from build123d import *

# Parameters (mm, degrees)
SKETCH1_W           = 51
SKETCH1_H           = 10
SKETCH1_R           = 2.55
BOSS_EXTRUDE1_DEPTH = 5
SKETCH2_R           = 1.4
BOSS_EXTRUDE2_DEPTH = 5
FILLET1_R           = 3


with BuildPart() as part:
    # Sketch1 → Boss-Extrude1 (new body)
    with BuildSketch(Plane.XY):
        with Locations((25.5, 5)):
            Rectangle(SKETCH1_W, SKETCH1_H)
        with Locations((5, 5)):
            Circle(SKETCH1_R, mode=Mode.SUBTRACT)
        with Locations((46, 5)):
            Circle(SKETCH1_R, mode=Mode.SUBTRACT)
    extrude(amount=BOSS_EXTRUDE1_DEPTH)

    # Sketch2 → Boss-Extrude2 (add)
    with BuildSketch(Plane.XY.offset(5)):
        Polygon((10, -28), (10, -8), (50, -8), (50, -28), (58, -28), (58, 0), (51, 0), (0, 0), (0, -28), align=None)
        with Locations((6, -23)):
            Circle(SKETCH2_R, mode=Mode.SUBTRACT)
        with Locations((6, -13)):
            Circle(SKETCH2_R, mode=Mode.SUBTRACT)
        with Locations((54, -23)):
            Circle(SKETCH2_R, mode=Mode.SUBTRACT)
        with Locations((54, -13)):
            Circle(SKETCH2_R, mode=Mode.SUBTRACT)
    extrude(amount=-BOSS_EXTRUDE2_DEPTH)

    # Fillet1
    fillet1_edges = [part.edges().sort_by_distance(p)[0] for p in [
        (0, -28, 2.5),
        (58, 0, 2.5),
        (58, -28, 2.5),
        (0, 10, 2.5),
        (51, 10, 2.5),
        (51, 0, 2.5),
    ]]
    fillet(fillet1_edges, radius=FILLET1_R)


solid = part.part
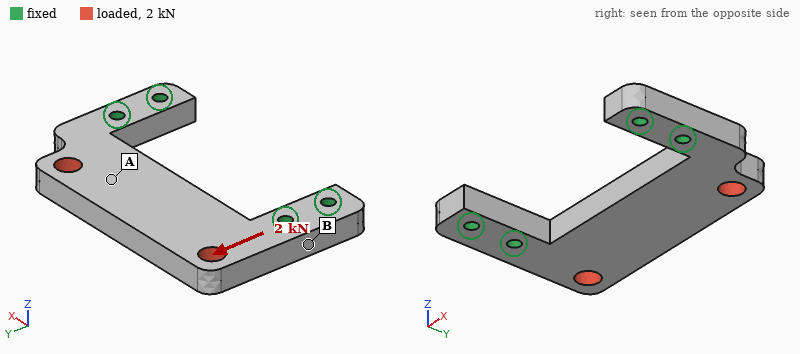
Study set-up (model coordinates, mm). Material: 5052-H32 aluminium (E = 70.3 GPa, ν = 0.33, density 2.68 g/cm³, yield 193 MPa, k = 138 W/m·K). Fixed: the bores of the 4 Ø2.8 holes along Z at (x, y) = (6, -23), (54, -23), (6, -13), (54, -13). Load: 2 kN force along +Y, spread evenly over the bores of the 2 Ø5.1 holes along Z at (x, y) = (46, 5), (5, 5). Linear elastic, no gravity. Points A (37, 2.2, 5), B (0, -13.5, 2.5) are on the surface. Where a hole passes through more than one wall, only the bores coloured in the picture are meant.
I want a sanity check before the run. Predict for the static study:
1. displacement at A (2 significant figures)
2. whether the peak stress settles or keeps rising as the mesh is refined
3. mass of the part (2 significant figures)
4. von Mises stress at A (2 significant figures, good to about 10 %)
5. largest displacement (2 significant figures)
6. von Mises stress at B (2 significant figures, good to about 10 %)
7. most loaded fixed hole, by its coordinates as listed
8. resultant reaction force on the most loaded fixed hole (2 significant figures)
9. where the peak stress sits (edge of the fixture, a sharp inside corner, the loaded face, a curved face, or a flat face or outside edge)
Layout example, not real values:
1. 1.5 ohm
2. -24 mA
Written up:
1. 9.1 µm
2. keeps rising
3. 17 g
4. 8.5 MPa
5. 11 µm
6. 17 MPa
7. (6, -13)
8. 1.1 kN
9. edge of the fixture
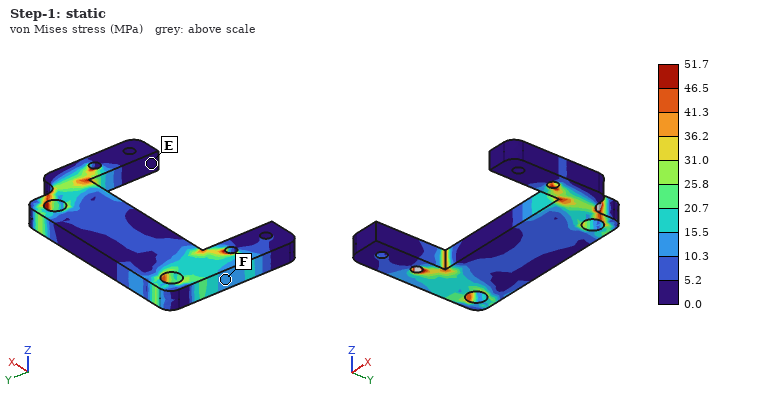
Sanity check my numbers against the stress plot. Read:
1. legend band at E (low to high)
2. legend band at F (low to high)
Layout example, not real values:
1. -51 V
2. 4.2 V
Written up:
1. 0.0 to 5.2 MPa
2. 10.3 to 15.5 MPa
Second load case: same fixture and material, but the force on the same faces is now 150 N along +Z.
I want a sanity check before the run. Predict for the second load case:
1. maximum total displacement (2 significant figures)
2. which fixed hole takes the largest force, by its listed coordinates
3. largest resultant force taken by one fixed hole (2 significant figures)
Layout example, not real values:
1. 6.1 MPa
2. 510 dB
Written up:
1. 34 µm
2. (6, -13)
3. 120 N
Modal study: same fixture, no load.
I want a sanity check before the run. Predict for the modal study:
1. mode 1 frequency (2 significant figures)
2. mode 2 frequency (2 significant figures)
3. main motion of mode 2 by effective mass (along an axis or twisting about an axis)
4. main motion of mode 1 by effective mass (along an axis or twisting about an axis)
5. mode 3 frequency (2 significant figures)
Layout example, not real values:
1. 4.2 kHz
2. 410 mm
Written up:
1. 4200 Hz
2. 9600 Hz
3. twisting about Y
4. along Z
5. 12 kHz
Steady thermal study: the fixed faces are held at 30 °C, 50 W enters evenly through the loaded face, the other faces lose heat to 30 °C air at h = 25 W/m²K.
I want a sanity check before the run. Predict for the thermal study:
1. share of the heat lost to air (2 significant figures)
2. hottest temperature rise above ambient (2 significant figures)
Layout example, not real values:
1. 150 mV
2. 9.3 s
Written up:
1. 5.8 %
2. 67 K
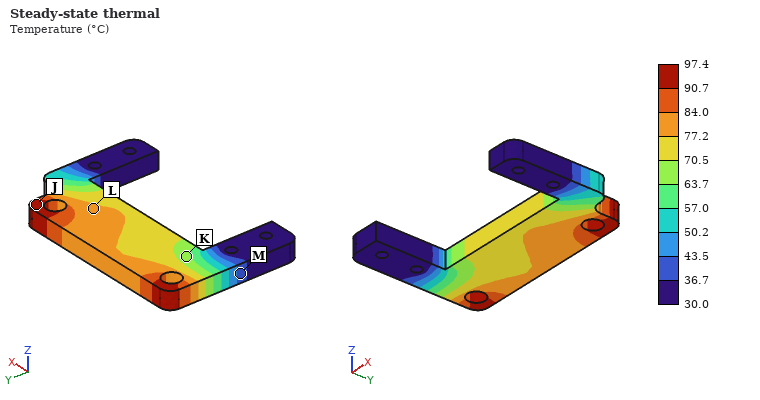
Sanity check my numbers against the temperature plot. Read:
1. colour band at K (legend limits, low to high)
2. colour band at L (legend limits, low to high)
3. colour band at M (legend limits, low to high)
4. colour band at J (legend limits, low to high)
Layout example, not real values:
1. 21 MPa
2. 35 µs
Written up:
1. 63.7 to 70.5 °C
2. 77.2 to 84.0 °C
3. 36.7 to 43.5 °C
4. 90.7 to 97.4 °C
